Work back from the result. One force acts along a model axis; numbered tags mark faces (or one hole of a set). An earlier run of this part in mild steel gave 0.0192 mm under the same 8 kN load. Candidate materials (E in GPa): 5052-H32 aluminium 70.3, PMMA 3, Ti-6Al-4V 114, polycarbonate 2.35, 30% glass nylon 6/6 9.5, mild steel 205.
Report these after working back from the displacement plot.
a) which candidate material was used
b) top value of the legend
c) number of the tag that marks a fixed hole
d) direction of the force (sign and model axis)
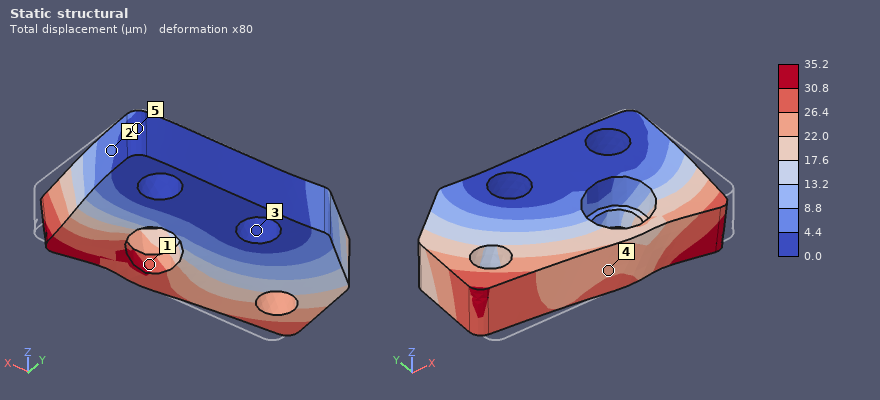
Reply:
Ti-6Al-4V
35.2 µm
3
-X
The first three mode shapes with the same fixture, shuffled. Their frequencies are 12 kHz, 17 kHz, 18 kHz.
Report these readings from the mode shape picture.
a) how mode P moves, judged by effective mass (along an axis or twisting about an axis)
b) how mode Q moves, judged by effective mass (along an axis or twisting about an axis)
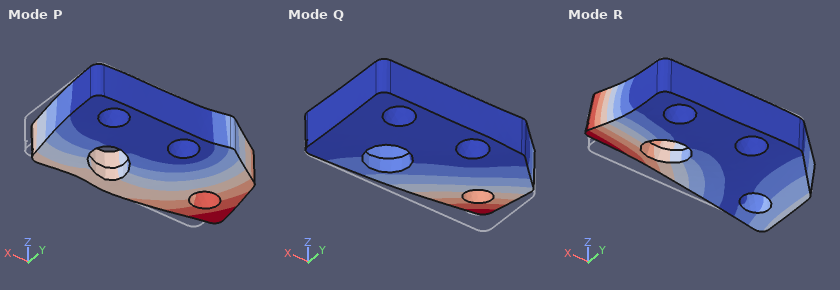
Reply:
along X
along Z
